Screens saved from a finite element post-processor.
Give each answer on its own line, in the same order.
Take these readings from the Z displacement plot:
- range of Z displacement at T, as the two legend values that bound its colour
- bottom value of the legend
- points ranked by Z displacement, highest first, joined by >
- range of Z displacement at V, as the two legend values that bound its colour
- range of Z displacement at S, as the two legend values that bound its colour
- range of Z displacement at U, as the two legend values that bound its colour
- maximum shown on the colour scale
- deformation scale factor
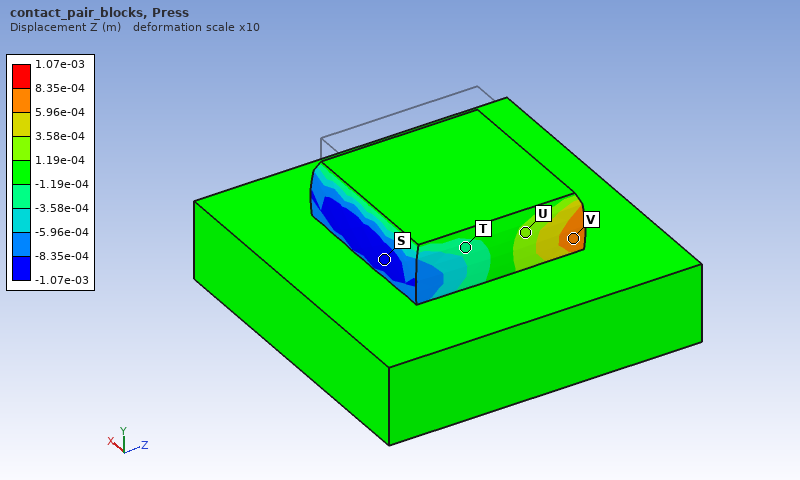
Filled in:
-3.58e-04 to -1.19e-04 m
-1.07e-03 m
V > U > T > S
5.96e-04 to 8.35e-04 m
-1.07e-03 to -8.35e-04 m
1.19e-04 to 3.58e-04 m
1.07e-03 m
10
